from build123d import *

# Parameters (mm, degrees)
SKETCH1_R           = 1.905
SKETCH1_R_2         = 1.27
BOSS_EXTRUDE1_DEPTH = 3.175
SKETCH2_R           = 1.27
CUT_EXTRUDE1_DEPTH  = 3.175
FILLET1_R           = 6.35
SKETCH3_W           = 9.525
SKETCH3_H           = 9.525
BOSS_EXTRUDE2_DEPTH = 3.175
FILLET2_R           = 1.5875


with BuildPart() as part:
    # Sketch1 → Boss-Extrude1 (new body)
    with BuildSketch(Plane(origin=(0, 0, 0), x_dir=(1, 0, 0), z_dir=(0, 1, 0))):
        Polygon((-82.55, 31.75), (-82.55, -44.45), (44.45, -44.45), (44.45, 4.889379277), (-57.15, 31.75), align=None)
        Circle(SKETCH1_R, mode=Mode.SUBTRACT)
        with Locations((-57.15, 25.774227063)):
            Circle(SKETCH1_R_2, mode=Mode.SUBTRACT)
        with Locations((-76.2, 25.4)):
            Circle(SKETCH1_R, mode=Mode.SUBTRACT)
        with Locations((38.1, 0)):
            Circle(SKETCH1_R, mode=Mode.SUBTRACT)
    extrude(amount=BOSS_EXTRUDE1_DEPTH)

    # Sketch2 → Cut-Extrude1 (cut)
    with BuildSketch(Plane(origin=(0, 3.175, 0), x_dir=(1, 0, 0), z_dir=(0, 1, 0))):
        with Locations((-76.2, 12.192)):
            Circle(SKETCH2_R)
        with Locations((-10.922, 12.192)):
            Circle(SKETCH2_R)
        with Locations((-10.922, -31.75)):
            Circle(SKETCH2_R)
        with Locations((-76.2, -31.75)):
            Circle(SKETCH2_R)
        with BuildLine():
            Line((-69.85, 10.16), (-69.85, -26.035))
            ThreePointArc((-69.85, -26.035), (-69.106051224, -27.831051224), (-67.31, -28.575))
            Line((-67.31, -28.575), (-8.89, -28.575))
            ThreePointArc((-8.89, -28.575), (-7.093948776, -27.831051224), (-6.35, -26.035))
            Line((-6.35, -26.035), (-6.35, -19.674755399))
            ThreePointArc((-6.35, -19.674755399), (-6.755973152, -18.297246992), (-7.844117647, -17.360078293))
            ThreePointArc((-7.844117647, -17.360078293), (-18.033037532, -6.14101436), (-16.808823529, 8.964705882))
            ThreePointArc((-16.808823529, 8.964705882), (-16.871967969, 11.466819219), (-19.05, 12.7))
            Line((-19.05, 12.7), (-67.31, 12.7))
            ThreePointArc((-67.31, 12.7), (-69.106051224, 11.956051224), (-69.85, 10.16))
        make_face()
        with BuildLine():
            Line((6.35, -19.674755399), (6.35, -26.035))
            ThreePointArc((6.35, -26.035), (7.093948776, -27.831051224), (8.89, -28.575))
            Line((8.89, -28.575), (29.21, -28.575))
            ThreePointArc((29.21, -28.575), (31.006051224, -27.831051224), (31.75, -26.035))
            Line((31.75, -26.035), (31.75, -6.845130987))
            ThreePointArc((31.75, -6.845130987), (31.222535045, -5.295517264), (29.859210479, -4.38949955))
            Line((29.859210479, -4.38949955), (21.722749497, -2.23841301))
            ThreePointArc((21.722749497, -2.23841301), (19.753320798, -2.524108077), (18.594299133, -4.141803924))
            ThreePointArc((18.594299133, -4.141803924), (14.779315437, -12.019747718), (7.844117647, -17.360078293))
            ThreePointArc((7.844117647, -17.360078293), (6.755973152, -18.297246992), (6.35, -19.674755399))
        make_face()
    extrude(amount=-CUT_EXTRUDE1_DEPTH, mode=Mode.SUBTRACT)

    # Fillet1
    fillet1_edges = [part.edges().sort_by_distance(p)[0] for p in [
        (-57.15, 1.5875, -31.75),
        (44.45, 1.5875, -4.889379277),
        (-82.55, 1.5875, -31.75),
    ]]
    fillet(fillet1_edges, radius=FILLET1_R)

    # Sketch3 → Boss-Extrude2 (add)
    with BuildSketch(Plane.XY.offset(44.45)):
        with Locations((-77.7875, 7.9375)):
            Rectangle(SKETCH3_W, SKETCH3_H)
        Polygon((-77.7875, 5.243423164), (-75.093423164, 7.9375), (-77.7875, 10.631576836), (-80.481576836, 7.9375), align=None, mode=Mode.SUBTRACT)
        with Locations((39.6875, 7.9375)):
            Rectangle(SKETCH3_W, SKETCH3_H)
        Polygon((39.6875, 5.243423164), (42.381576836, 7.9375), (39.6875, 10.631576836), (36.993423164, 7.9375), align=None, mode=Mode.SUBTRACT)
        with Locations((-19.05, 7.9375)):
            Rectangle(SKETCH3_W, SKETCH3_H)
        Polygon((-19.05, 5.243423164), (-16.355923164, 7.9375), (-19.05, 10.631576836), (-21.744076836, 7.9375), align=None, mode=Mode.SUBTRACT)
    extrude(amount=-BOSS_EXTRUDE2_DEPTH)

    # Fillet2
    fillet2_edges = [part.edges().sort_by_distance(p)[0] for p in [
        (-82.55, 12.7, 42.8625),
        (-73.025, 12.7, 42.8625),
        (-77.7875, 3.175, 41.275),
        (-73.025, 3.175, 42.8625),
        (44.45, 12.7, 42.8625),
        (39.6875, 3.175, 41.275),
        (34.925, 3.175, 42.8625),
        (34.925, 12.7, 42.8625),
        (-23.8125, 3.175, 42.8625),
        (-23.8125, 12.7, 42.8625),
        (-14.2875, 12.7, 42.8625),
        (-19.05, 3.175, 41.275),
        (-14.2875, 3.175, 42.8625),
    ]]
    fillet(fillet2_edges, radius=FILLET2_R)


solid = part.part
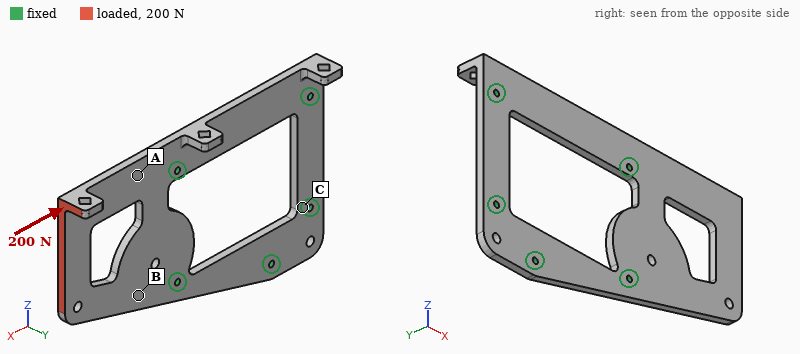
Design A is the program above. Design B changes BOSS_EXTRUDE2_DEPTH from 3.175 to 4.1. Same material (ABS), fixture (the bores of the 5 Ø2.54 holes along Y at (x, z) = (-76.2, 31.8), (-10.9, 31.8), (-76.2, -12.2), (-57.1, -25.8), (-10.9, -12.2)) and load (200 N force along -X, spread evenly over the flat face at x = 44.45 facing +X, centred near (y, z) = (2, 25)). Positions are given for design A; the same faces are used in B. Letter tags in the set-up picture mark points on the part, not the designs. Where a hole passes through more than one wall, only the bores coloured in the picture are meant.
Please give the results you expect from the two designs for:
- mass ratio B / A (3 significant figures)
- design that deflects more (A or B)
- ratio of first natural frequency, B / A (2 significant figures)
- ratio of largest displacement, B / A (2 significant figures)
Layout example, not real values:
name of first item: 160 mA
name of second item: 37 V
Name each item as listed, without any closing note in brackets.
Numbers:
mass ratio B / A: 1.01
design that deflects more: B
ratio of first natural frequency, B / A: 0.99
ratio of largest displacement, B / A: 1.2
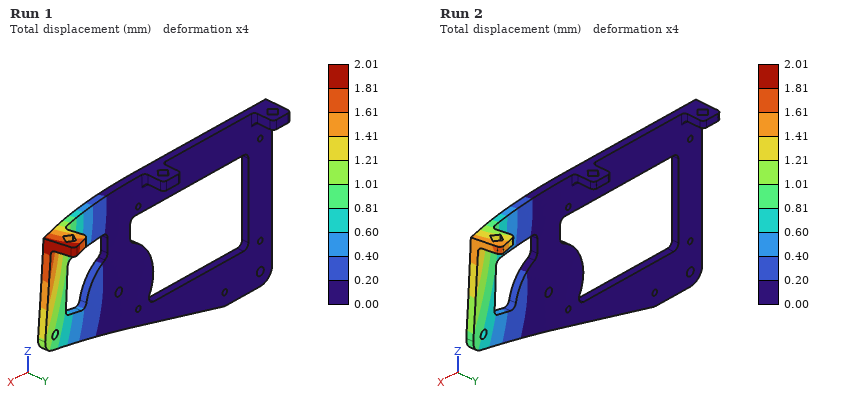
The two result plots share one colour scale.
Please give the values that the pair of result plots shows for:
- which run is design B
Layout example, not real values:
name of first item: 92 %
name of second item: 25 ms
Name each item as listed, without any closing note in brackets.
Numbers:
which run is design B: Run 1
